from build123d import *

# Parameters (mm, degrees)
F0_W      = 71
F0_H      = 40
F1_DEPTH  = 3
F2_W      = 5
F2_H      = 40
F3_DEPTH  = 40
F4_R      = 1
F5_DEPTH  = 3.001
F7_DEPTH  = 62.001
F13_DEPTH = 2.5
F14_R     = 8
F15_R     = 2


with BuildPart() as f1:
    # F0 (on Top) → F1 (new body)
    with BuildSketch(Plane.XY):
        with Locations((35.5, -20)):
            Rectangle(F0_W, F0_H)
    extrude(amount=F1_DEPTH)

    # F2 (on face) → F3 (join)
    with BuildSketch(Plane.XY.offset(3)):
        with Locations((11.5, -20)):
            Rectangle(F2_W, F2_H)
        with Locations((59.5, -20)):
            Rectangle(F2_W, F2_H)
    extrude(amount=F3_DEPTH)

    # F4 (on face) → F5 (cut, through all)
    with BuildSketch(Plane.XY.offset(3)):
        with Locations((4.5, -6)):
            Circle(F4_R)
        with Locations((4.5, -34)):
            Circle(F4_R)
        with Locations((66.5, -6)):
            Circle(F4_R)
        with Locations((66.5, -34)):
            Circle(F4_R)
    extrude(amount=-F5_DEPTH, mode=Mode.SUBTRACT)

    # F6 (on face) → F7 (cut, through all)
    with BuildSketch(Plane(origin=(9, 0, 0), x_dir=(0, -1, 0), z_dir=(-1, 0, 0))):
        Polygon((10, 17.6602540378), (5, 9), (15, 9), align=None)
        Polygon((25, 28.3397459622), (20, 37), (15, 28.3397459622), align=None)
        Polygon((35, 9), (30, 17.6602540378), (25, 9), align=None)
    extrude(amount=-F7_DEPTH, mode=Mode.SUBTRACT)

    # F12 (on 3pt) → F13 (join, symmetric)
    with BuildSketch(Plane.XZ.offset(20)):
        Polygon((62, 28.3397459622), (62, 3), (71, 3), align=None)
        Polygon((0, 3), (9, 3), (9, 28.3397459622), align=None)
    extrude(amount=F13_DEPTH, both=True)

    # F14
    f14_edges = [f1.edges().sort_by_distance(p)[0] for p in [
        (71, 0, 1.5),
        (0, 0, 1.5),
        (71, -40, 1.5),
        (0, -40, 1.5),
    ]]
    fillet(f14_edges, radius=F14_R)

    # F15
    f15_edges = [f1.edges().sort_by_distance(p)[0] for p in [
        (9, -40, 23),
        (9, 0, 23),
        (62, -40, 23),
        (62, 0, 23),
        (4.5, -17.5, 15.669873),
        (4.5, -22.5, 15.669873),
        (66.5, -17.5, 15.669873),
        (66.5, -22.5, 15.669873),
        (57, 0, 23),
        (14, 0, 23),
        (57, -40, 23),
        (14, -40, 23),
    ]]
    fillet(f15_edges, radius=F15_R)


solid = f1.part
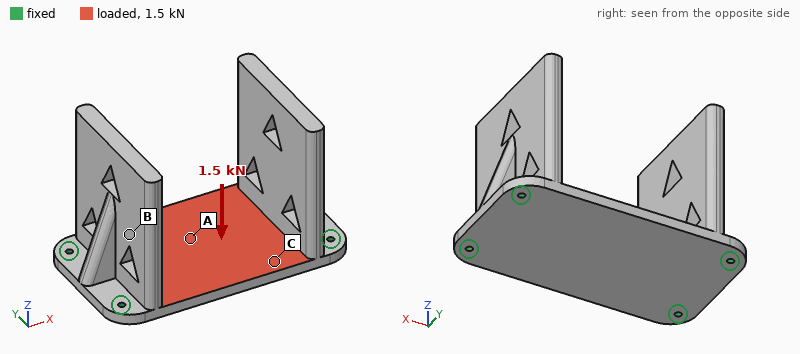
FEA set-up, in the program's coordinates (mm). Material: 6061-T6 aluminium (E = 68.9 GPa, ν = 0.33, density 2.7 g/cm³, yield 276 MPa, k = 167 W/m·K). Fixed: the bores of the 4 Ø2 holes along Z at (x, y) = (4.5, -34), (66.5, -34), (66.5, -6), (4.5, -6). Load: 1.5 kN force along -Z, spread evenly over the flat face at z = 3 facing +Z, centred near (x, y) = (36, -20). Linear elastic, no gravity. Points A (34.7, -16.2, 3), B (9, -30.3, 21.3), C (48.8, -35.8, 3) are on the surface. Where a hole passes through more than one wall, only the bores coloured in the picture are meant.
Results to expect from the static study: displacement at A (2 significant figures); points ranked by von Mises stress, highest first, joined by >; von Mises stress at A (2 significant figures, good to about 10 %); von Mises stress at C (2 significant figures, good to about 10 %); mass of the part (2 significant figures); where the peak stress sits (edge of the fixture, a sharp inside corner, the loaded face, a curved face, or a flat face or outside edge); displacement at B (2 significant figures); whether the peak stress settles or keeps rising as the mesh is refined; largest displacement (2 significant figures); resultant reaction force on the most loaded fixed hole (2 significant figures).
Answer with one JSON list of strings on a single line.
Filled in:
["0.23 mm", "A > C > B", "85 MPa", "46 MPa", "64 g", "edge of the fixture", "0.19 mm", "keeps rising", "0.40 mm", "380 N"]
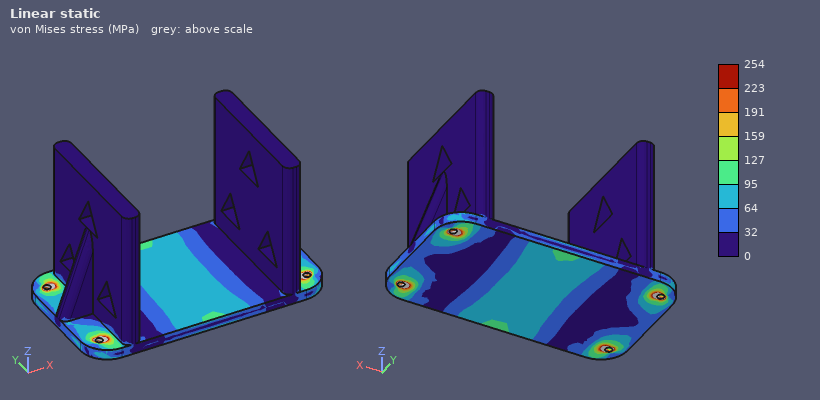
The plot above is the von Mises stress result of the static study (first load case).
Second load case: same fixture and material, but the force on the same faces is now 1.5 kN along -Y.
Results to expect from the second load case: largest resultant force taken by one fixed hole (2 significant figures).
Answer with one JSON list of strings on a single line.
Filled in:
["470 N"]
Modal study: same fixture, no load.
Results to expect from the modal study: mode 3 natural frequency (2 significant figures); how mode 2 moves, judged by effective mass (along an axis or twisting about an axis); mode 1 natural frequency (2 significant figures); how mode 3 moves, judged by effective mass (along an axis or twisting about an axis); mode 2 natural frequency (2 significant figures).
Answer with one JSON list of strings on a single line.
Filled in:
["4000 Hz", "along X", "1300 Hz", "along Y", "1700 Hz"]
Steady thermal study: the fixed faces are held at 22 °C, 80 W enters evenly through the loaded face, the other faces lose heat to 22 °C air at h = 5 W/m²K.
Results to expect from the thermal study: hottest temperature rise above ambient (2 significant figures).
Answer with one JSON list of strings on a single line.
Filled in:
["47 K"]
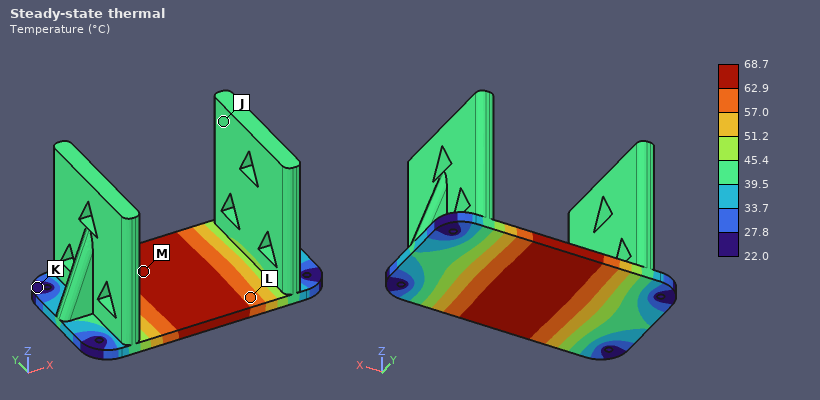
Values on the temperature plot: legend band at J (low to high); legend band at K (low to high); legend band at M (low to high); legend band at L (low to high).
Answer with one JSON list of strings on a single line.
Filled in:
["39.5 to 45.4 °C", "22.0 to 27.8 °C", "62.9 to 68.7 °C", "57.0 to 62.9 °C"]
